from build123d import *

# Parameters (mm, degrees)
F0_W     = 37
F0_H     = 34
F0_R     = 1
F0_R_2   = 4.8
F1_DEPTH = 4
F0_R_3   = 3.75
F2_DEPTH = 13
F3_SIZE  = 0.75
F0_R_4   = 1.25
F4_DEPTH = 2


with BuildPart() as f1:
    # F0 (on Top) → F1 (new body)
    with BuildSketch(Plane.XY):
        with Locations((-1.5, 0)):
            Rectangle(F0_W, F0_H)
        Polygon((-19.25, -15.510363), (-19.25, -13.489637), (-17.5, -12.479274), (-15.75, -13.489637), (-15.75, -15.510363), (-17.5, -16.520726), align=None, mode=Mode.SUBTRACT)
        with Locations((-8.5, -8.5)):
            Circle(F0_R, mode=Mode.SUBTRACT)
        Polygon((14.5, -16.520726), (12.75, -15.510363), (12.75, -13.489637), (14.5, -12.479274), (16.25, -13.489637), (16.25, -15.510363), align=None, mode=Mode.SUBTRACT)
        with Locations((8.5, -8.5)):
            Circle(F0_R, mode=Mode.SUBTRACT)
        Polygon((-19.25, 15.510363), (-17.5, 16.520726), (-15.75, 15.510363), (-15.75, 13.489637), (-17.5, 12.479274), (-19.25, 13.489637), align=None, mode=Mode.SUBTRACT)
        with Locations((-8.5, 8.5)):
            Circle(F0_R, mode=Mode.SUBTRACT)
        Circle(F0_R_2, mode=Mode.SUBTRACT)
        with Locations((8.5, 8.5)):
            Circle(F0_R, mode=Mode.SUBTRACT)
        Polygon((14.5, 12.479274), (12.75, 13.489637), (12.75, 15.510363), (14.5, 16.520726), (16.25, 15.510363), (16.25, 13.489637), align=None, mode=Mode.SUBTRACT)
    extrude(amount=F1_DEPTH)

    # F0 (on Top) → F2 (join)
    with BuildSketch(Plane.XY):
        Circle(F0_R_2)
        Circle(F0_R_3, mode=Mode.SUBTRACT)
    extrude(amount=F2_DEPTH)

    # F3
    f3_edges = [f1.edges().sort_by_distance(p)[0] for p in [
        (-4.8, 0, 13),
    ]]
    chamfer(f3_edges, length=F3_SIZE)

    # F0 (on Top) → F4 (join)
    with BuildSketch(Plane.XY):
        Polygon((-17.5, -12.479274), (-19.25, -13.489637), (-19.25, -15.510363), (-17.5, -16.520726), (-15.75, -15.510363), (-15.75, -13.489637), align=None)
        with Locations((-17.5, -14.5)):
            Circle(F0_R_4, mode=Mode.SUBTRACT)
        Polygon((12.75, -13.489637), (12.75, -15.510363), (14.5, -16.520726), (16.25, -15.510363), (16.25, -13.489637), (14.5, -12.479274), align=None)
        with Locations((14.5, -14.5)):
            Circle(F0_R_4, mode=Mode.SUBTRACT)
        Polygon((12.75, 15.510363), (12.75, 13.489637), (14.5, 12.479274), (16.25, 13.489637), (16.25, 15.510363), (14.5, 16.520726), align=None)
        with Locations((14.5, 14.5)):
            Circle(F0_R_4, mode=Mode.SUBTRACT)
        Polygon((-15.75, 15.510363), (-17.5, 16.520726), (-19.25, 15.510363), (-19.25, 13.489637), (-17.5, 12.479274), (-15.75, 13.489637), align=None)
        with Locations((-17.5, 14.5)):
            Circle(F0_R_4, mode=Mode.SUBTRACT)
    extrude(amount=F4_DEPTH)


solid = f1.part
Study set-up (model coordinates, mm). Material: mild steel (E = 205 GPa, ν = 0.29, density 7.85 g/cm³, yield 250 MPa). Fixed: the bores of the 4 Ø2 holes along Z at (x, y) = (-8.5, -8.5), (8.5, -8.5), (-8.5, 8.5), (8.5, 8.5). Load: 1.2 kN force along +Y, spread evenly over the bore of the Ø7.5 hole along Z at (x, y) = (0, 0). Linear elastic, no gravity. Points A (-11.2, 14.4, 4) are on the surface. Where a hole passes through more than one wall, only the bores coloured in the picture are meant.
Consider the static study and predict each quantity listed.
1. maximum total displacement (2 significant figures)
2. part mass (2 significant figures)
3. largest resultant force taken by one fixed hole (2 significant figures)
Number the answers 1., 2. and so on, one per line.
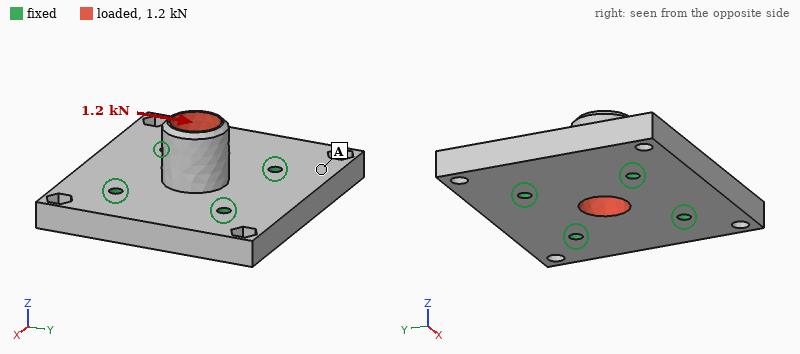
1. 9.7 µm
2. 39 g
3. 360 N
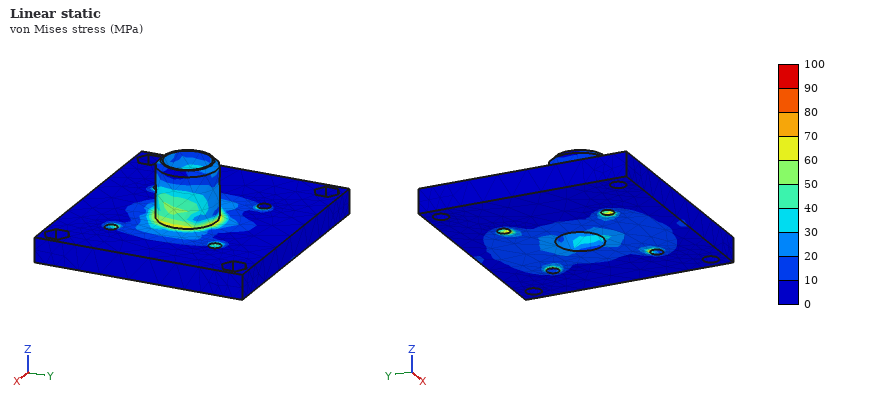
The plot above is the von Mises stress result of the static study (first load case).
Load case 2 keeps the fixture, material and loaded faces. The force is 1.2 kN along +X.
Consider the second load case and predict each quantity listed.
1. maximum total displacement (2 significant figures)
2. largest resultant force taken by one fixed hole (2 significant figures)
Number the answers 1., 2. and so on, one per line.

1. 9.8 µm
2. 360 N
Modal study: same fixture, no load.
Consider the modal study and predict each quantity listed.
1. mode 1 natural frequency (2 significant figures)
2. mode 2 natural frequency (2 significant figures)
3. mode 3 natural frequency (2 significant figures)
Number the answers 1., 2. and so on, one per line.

1. 20 kHz
2. 24 kHz
3. 29 kHz
